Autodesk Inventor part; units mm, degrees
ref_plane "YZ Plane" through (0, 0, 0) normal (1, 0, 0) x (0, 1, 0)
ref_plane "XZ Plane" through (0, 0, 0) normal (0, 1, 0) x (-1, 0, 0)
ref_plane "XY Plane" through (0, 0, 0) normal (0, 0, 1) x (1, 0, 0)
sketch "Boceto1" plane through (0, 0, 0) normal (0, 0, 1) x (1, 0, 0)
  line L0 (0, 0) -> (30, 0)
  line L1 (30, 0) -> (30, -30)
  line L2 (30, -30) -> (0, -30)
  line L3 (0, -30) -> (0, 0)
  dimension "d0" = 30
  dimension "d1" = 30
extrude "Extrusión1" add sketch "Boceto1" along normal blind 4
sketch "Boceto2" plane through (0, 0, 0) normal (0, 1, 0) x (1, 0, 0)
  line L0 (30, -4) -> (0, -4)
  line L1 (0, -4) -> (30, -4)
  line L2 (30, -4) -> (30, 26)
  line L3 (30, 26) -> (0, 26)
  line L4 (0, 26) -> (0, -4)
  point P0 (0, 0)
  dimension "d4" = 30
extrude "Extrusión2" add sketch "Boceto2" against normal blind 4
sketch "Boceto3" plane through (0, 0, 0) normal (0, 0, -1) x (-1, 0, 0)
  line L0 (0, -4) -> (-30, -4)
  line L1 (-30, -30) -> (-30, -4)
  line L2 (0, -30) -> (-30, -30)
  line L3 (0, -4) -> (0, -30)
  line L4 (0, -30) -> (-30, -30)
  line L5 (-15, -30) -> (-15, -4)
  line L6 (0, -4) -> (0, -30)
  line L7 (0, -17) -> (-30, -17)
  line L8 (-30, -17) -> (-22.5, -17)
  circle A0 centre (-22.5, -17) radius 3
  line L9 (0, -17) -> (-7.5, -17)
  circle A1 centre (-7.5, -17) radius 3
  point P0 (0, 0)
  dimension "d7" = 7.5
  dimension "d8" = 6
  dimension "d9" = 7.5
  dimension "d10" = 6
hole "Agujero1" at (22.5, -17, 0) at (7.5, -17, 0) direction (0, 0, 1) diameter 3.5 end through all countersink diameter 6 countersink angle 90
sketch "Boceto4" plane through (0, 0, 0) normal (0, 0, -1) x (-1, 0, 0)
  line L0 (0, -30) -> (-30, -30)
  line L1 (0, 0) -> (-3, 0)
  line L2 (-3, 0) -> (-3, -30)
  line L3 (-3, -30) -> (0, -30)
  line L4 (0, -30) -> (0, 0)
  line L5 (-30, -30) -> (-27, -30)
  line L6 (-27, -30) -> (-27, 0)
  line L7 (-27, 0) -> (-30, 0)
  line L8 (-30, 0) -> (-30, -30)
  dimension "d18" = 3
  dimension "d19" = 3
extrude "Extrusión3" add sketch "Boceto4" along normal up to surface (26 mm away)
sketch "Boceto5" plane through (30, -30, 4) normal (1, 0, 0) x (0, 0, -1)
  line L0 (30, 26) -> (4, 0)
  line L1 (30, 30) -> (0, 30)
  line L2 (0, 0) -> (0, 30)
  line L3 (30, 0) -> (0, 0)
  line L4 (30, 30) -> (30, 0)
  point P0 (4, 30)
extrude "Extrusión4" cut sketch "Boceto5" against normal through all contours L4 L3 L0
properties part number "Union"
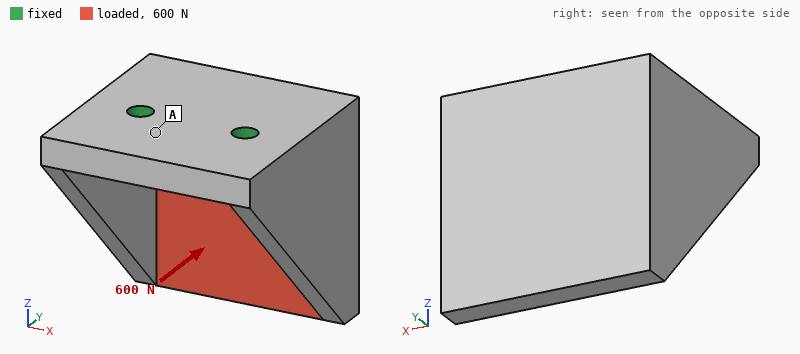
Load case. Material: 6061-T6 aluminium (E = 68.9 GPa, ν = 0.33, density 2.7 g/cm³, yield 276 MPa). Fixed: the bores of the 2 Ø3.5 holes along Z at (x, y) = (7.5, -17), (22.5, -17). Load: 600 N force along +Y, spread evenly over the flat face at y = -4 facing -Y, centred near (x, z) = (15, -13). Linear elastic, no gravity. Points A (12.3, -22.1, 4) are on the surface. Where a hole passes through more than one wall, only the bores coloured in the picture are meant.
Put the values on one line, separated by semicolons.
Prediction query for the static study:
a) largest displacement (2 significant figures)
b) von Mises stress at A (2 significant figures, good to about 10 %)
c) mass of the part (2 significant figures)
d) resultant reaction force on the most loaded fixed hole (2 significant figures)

0.13 mm; 20 MPa; 23 g; 300 N
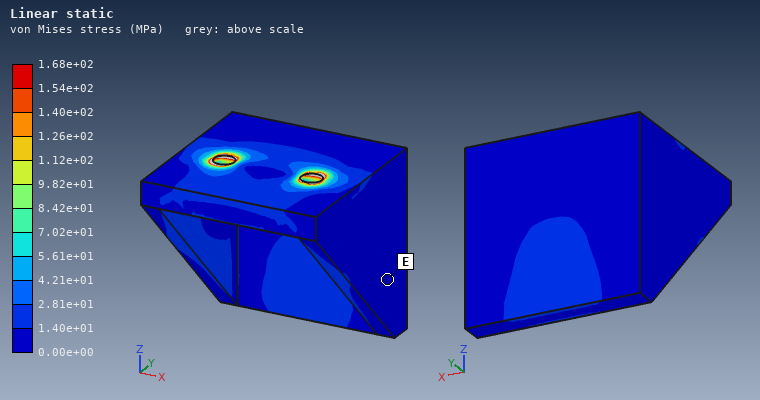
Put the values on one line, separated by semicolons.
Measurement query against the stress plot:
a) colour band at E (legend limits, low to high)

0.00e+00 to 1.40e+01 MPa
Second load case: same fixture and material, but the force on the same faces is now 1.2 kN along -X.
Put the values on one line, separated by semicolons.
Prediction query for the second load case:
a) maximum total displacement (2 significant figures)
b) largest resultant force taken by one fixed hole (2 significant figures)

0.17 mm; 1.4 kN
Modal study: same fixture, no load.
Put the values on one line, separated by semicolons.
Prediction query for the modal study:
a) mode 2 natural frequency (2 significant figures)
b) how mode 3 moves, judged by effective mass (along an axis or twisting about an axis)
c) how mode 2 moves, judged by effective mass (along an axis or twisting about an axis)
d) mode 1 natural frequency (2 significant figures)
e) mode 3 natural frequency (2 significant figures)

4600 Hz; along X; along X; 3400 Hz; 12 kHz
